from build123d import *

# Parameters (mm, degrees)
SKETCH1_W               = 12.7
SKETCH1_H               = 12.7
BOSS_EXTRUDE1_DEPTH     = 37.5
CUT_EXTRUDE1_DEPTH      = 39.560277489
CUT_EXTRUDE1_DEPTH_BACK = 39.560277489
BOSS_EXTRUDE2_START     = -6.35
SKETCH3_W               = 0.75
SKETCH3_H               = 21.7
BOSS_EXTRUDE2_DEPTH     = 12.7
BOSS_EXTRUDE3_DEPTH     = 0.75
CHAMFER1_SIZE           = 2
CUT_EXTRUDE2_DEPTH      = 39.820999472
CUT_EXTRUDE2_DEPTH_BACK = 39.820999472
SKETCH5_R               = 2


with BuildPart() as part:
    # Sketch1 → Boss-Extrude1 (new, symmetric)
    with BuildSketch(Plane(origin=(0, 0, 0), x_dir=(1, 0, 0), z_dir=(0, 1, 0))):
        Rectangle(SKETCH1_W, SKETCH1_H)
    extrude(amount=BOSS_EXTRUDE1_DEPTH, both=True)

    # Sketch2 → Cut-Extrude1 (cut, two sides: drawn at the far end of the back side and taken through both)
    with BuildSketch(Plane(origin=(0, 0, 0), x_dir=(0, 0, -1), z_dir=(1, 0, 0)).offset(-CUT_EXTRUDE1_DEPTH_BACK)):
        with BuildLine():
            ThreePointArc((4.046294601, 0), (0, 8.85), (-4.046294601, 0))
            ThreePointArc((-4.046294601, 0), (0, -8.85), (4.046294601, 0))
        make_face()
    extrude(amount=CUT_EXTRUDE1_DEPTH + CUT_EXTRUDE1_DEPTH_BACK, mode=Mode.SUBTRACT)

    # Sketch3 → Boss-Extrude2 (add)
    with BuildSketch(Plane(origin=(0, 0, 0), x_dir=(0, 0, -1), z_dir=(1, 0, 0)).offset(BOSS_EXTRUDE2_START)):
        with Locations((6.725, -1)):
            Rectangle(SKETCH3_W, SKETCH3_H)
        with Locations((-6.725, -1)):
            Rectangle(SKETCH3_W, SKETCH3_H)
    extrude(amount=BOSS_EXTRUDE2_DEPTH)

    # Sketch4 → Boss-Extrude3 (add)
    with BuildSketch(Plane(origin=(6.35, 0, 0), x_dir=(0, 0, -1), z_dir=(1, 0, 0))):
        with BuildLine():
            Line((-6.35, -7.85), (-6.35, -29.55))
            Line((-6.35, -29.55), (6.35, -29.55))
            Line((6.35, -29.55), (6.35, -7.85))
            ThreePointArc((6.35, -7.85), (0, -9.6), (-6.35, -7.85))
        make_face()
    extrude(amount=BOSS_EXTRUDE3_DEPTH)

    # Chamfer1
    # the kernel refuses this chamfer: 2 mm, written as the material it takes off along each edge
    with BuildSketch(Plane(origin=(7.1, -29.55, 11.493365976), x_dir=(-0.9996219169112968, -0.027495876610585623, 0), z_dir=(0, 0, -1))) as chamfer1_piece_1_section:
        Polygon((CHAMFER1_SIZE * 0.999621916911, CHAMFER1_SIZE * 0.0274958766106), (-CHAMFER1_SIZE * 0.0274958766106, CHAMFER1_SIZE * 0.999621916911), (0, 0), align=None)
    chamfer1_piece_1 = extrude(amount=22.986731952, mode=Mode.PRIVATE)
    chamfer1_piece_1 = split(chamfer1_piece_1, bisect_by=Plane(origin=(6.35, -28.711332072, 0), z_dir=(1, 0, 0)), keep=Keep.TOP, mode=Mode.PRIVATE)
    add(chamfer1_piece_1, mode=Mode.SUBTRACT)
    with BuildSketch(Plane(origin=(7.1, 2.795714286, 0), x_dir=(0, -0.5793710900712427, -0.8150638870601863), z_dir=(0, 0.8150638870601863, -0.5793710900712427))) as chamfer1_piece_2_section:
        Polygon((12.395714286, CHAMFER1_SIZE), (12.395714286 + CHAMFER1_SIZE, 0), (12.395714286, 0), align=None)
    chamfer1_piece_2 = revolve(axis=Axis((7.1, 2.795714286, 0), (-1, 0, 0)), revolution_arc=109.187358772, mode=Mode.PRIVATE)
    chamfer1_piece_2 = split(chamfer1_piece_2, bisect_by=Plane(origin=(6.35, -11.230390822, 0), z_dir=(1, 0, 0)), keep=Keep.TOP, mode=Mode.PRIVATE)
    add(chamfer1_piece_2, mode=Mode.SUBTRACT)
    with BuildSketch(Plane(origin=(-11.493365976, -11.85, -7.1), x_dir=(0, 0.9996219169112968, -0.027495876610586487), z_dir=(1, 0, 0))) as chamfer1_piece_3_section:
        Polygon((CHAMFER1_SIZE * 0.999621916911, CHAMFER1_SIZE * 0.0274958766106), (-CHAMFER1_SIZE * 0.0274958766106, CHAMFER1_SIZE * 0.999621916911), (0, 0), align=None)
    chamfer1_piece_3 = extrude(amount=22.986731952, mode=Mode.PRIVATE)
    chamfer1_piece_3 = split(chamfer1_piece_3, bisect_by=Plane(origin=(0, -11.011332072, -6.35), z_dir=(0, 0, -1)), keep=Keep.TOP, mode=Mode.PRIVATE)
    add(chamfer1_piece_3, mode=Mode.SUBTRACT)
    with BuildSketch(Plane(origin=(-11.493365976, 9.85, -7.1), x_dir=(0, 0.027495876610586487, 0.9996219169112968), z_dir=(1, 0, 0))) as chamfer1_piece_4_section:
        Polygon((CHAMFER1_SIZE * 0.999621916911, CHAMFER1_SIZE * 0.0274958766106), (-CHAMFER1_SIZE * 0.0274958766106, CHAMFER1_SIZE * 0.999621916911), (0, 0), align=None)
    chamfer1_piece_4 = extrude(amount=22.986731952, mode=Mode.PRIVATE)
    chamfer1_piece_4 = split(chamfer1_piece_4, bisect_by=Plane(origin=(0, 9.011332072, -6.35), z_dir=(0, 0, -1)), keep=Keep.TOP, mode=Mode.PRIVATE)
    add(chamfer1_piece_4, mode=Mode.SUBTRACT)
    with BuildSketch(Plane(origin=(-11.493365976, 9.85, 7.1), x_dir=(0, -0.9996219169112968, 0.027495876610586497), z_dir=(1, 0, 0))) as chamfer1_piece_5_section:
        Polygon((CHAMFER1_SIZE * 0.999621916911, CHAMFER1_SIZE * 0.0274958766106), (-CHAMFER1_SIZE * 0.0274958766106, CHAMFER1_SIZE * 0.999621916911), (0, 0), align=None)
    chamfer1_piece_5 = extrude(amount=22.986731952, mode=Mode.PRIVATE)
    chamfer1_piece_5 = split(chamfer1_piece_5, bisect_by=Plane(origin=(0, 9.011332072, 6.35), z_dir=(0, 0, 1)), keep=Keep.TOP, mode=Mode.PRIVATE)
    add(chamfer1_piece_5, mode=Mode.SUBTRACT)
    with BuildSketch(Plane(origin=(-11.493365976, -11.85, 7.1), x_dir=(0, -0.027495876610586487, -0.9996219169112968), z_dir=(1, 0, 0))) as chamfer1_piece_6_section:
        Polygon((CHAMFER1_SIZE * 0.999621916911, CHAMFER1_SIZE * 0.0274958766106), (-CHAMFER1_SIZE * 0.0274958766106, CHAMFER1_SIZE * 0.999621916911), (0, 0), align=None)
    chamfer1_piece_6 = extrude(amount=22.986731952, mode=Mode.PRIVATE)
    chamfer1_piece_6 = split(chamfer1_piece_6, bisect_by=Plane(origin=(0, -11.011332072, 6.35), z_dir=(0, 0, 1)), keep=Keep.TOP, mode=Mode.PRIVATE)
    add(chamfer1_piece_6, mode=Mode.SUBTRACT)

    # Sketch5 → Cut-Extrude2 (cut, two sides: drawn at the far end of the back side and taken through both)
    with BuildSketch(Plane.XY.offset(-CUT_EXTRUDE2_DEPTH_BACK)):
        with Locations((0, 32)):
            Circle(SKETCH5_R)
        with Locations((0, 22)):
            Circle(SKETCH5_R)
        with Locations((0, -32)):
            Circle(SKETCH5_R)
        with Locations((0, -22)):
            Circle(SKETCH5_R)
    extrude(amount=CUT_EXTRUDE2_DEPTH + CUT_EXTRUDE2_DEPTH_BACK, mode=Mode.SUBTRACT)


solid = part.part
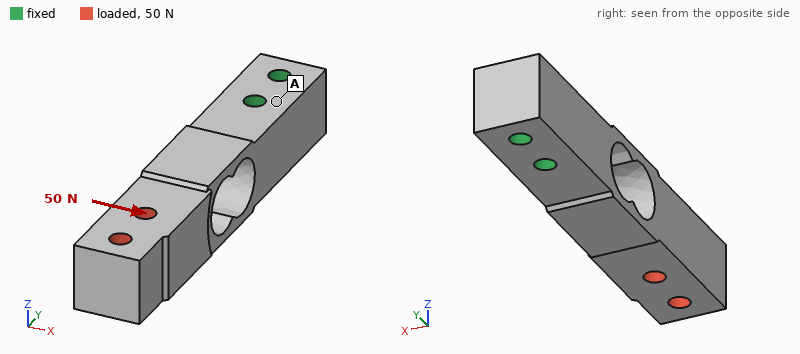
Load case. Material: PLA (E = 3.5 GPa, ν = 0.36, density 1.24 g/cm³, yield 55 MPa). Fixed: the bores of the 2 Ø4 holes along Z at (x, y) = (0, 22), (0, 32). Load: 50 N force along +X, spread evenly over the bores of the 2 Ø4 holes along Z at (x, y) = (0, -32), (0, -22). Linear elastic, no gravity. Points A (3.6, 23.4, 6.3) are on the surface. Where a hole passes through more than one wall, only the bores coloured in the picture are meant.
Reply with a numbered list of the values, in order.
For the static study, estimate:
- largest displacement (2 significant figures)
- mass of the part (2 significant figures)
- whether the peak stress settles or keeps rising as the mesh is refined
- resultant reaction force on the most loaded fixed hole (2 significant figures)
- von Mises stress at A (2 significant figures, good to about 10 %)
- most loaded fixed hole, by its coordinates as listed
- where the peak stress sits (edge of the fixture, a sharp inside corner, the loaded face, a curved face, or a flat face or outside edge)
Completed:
1. 0.81 mm
2. 12 g
3. keeps rising
4. 160 N
5. 3.2 MPa
6. (0, 22)
7. a sharp inside corner
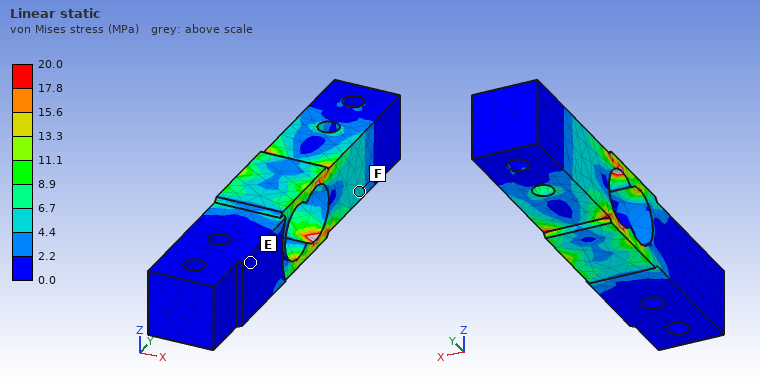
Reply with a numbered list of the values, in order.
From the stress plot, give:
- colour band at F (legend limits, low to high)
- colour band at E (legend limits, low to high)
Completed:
1. 4.4 to 6.7 MPa
2. 0.0 to 2.2 MPa
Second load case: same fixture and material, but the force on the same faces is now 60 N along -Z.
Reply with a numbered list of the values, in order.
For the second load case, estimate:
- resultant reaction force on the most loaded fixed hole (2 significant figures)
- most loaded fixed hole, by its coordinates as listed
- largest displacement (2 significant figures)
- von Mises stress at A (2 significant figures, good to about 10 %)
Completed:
1. 92 N
2. (0, 22)
3. 0.81 mm
4. 3.1 MPa
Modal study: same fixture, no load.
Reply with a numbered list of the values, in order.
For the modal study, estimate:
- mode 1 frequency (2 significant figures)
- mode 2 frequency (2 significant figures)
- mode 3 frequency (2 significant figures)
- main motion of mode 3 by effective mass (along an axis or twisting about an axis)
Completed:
1. 650 Hz
2. 660 Hz
3. 2600 Hz
4. twisting about Y
